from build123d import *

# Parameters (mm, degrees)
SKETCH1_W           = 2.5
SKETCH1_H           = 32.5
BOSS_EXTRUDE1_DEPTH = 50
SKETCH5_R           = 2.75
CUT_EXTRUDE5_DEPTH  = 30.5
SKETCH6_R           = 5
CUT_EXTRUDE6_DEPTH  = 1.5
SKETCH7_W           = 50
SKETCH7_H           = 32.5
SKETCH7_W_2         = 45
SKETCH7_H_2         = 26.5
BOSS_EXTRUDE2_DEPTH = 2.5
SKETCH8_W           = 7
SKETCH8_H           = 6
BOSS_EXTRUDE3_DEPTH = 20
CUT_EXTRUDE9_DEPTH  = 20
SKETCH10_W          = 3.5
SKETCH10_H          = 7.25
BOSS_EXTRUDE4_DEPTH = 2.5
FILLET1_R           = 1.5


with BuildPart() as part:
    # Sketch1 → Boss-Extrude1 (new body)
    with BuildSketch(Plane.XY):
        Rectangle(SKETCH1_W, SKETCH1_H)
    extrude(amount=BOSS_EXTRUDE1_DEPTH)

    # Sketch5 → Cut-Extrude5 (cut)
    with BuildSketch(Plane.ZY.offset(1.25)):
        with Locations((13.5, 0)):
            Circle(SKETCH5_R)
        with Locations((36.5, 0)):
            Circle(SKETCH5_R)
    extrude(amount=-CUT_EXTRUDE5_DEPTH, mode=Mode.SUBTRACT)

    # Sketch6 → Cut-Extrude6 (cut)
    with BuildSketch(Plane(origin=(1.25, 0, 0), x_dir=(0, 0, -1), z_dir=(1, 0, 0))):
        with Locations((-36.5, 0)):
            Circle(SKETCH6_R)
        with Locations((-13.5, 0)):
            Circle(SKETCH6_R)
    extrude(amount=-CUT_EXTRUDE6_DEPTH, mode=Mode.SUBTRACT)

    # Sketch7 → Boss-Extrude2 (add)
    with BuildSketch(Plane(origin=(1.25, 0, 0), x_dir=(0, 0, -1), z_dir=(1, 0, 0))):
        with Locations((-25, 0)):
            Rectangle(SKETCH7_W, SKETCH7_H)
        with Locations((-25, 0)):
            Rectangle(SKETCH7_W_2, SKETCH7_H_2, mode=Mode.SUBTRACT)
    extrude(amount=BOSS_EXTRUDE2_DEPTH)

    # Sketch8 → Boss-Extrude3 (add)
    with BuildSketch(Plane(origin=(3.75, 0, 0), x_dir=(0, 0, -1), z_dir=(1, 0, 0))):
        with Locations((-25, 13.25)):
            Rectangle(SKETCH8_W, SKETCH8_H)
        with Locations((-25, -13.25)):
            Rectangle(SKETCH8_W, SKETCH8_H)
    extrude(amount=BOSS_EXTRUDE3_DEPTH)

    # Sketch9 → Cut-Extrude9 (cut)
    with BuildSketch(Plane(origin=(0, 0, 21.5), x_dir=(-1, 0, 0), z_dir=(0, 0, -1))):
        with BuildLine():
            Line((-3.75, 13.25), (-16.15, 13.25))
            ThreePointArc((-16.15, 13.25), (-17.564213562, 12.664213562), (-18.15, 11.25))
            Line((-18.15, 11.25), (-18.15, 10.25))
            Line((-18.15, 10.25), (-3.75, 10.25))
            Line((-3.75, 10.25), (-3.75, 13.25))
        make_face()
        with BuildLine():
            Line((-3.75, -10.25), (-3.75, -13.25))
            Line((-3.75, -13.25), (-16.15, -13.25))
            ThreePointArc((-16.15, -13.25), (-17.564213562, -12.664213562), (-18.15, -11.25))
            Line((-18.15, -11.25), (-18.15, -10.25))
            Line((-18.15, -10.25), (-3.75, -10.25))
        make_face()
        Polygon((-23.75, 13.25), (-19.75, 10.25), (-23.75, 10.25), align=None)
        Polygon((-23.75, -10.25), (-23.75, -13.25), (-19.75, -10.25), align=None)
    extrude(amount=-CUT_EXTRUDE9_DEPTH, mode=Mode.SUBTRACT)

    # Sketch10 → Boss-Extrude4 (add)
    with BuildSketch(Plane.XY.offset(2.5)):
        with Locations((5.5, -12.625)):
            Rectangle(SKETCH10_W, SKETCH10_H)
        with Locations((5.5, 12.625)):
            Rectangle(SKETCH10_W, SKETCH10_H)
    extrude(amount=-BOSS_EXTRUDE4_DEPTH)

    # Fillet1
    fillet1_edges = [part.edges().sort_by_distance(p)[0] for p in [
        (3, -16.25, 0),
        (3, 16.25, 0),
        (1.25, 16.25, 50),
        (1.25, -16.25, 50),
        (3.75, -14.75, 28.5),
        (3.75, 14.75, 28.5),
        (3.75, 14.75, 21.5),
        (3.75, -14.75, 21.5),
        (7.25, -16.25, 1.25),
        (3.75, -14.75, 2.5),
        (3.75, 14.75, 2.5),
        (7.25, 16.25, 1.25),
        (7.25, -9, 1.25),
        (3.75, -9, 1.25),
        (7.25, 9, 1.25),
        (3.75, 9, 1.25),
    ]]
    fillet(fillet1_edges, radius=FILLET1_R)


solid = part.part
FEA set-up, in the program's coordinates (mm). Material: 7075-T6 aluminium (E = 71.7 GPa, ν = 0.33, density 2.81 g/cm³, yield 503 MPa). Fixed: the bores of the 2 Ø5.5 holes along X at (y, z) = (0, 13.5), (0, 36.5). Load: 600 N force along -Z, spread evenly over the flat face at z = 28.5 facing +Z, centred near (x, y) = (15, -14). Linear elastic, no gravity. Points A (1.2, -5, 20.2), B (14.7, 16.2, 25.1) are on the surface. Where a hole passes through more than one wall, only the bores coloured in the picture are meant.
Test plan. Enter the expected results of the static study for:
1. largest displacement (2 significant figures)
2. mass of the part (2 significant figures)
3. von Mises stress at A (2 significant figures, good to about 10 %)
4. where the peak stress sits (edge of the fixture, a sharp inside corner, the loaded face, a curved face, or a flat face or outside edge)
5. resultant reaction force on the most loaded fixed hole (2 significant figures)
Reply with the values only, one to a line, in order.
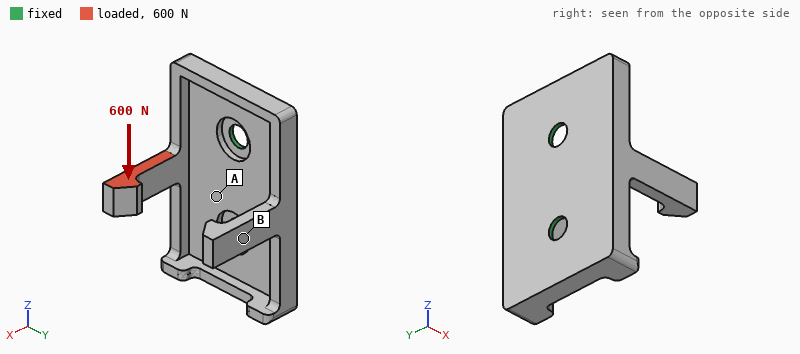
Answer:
0.48 mm
17 g
120 MPa
a curved face
620 N
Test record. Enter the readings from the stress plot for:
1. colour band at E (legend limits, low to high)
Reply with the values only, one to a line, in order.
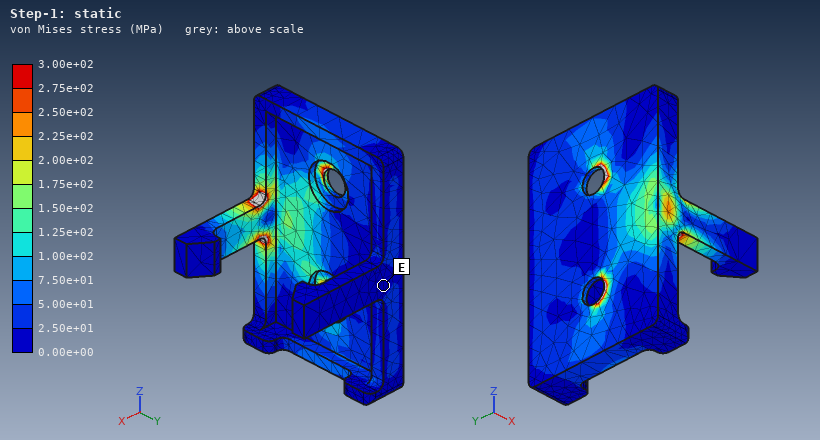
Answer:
0.00e+00 to 2.50e+01 MPa
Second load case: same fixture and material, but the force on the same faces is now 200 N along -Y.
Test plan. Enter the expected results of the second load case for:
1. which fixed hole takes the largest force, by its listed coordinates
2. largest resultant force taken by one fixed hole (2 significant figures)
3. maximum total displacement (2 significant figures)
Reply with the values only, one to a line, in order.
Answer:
(0, 36.5)
150 N
0.75 mm
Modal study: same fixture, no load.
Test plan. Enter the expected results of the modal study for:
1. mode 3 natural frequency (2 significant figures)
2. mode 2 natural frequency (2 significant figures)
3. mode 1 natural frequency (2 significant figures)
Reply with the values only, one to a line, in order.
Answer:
4000 Hz
2900 Hz
2000 Hz
